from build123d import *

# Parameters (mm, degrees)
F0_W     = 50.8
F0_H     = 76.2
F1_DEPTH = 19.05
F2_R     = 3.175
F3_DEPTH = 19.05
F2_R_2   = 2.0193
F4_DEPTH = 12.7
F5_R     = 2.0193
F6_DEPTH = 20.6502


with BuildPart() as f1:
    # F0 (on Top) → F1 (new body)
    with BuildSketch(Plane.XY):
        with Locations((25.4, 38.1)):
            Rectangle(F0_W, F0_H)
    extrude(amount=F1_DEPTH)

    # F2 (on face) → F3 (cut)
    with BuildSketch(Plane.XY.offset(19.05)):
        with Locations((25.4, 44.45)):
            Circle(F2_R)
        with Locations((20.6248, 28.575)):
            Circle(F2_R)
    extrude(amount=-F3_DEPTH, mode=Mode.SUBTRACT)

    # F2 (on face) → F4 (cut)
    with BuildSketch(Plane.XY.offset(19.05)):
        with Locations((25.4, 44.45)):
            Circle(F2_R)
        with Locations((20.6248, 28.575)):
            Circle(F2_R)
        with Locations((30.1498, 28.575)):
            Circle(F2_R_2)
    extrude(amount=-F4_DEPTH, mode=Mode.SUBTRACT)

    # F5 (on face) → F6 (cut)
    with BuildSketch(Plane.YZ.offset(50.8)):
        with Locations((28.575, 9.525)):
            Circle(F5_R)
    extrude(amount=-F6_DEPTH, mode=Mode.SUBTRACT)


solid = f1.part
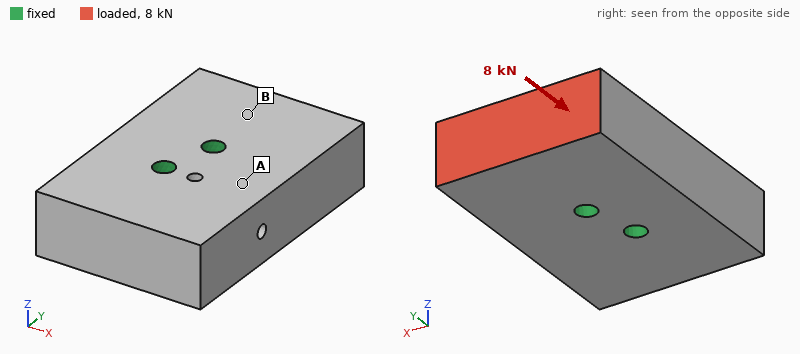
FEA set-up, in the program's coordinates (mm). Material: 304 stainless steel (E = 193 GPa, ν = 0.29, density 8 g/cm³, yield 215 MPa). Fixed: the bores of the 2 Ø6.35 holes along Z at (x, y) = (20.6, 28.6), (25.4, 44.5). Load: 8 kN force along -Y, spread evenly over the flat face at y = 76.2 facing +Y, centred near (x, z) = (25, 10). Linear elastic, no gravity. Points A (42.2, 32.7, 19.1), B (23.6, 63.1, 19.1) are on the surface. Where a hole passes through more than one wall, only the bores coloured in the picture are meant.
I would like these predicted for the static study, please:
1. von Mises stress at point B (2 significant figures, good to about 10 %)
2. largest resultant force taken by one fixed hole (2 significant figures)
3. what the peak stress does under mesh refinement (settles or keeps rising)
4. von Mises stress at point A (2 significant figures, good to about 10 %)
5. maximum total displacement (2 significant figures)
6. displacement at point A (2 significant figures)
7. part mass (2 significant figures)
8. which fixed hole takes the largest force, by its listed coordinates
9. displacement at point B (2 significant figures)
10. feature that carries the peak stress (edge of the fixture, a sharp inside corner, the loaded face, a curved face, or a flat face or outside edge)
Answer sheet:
11 MPa
5.6 kN
keeps rising
3.8 MPa
2.6 µm
0.88 µm
580 g
(25.4, 44.5)
1.2 µm
edge of the fixture
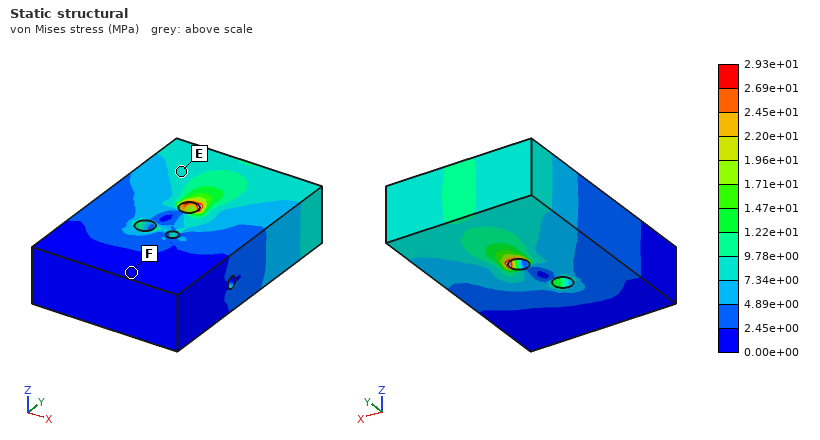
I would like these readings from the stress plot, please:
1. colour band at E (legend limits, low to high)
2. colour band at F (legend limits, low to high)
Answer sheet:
7.34e+00 to 9.78e+00 MPa
0.00e+00 to 2.45e+00 MPa
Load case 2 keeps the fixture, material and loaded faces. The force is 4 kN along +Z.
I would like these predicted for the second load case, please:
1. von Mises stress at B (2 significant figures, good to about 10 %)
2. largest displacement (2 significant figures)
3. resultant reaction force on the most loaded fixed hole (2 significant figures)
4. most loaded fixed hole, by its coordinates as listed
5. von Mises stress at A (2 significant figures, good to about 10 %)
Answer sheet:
17 MPa
14 µm
5.6 kN
(25.4, 44.5)
12 MPa
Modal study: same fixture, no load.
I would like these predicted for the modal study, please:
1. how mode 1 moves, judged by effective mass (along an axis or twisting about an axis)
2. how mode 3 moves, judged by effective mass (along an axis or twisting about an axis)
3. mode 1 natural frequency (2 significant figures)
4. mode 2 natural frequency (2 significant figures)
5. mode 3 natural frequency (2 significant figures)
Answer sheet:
twisting about Z
along Z
8600 Hz
9100 Hz
10 kHz
